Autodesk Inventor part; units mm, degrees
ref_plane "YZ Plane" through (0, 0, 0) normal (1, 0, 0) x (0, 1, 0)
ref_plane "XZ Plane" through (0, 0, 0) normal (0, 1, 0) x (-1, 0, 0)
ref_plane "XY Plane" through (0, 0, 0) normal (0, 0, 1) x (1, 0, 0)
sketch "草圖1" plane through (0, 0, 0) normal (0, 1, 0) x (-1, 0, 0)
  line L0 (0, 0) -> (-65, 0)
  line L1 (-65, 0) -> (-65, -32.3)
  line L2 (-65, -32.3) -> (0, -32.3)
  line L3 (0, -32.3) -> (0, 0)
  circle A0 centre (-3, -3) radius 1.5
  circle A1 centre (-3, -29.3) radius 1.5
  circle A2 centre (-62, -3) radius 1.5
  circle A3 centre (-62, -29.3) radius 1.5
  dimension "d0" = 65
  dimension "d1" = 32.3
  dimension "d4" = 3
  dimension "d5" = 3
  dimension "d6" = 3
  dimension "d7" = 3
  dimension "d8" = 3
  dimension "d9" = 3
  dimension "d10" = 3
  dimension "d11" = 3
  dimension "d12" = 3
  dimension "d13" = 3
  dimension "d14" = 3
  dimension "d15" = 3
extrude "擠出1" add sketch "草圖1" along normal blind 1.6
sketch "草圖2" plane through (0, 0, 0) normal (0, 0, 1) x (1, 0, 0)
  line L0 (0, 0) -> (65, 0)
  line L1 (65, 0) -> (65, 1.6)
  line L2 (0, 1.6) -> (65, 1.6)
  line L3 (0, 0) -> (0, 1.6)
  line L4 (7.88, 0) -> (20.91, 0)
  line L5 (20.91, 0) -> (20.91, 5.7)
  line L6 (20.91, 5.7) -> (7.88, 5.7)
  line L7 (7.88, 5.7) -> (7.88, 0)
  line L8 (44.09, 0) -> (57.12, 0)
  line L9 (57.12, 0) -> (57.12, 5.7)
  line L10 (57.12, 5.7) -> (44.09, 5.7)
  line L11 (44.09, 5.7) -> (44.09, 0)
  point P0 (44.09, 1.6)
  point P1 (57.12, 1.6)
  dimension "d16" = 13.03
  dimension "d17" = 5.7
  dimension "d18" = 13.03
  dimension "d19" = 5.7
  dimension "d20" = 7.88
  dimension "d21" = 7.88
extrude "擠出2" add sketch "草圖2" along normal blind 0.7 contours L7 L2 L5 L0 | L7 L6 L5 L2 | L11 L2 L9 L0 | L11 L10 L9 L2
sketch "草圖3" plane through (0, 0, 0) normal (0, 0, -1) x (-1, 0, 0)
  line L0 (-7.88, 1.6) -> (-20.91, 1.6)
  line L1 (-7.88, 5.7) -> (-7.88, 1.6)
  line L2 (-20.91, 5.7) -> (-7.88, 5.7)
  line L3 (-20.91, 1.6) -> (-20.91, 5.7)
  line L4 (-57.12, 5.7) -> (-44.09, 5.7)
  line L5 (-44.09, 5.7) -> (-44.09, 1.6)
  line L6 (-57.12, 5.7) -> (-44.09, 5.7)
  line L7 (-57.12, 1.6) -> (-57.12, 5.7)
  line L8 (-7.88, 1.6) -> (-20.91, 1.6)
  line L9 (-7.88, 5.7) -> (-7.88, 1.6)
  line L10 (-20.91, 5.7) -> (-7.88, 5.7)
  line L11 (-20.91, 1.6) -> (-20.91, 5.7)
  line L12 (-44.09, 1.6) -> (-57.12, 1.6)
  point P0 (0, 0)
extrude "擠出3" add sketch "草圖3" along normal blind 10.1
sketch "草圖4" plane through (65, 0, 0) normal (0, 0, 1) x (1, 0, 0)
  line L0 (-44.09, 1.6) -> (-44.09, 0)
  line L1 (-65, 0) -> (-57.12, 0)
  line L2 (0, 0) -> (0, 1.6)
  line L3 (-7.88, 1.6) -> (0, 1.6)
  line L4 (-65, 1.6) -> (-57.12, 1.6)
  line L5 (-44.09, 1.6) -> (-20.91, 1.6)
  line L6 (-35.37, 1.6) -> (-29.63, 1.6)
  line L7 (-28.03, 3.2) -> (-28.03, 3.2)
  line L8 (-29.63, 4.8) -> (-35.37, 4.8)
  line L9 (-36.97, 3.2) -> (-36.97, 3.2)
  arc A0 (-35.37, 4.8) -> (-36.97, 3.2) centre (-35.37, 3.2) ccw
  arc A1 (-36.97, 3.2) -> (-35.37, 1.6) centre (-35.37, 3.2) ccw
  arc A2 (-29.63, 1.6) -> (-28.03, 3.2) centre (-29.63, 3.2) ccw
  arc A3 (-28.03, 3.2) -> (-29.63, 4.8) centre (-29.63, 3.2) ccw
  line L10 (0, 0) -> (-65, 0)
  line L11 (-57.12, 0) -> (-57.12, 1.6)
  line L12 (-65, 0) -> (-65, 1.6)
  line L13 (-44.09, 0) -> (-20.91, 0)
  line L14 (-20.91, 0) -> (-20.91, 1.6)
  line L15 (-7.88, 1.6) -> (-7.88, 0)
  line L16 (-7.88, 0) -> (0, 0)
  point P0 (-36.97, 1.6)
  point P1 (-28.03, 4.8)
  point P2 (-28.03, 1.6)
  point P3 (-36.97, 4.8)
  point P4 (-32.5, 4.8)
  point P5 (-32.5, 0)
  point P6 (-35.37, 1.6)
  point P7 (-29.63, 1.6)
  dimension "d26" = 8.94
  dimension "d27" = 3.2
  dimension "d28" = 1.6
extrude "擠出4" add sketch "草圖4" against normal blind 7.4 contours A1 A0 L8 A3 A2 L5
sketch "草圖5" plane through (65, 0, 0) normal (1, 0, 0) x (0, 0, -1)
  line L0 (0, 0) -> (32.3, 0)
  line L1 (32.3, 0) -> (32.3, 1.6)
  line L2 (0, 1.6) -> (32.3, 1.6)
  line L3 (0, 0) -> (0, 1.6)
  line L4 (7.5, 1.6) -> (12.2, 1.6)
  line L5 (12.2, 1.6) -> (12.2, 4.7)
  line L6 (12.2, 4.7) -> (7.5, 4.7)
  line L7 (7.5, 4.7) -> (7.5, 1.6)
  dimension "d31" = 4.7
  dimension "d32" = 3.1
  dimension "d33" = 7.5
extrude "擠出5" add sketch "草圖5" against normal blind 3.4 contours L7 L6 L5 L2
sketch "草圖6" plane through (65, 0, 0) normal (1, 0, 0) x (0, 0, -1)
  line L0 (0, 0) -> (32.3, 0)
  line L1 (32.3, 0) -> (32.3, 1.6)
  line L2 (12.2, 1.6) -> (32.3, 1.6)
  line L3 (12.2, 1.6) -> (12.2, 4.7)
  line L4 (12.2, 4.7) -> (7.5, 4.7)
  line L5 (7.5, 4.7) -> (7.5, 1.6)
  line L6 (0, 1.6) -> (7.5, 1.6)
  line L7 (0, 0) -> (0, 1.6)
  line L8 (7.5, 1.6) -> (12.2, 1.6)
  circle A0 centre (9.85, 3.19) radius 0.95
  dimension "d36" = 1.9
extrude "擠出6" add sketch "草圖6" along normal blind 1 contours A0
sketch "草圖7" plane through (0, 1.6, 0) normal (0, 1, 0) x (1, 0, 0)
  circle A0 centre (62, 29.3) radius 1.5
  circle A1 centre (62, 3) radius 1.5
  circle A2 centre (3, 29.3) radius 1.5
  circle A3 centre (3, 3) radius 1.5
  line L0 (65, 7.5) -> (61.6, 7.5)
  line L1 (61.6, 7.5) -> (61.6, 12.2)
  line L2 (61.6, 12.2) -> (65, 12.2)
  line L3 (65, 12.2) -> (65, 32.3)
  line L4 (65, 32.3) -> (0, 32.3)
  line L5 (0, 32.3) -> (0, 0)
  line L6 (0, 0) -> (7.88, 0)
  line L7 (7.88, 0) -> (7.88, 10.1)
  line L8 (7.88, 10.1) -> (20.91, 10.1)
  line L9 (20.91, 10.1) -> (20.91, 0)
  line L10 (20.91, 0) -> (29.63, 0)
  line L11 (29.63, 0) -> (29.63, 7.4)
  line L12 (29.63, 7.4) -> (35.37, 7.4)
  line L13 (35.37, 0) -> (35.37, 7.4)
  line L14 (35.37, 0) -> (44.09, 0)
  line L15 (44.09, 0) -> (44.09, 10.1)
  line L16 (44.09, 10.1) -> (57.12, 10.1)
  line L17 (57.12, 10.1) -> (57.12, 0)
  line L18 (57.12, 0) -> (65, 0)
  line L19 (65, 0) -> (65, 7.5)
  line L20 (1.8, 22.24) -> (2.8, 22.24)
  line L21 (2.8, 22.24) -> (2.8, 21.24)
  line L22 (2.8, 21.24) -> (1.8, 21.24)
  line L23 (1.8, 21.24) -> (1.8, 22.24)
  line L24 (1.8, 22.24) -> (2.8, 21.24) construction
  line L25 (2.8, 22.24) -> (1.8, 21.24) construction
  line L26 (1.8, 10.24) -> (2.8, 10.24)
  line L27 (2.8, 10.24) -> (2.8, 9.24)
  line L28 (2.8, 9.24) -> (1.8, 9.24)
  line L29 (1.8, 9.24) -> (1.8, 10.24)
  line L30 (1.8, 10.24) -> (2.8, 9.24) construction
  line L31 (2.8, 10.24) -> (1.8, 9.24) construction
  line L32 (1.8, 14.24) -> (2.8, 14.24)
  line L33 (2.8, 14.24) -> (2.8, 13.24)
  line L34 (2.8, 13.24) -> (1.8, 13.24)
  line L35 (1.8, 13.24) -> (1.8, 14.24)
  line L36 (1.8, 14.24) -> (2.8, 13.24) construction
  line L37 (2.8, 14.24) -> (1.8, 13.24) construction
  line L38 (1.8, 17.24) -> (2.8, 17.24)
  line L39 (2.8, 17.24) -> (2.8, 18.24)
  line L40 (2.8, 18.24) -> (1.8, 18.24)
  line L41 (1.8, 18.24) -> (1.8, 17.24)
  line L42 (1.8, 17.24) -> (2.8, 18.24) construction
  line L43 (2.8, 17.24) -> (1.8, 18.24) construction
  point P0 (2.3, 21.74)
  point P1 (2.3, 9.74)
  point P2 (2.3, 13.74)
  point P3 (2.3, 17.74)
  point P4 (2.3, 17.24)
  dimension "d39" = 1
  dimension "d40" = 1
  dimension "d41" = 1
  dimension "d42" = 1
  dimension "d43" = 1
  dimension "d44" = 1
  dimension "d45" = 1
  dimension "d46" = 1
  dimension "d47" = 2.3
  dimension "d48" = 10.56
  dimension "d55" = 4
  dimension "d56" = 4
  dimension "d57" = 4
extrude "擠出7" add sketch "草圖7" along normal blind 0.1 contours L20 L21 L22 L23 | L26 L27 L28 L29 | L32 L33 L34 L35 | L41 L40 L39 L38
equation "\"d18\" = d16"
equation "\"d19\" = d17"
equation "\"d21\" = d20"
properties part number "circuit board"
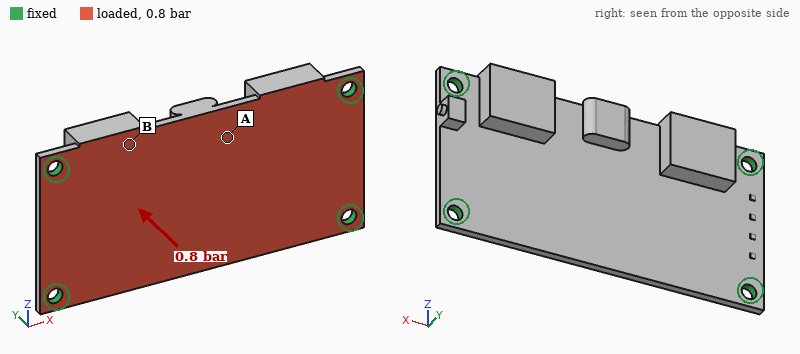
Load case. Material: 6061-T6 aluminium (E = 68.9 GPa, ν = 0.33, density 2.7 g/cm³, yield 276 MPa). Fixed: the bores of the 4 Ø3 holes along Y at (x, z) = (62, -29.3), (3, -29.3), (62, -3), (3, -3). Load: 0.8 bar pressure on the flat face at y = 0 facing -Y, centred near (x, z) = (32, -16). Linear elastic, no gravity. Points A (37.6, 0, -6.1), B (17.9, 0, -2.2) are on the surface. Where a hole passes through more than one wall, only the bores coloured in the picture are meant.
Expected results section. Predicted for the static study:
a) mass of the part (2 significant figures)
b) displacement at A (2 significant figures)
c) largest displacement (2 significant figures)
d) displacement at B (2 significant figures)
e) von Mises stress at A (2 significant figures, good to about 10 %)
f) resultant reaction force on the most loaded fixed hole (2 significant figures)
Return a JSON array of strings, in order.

["13 g", "0.095 mm", "0.12 mm", "0.056 mm", "26 MPa", "42 N"]
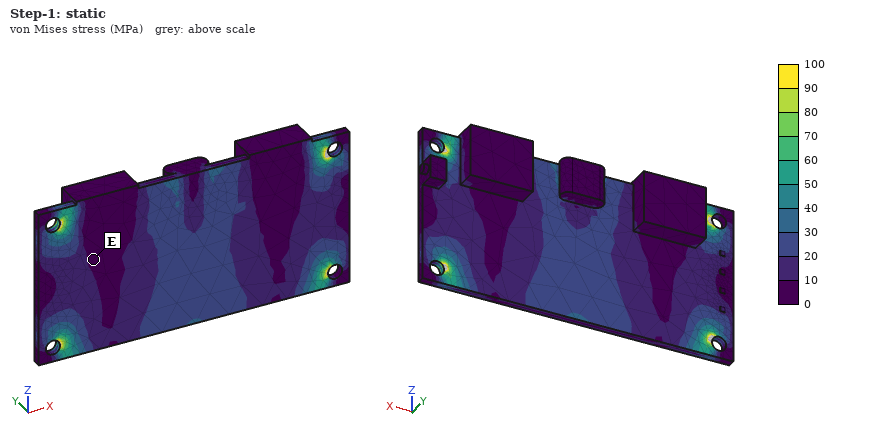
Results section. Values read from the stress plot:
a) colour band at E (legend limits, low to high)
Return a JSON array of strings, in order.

["0 to 10 MPa"]
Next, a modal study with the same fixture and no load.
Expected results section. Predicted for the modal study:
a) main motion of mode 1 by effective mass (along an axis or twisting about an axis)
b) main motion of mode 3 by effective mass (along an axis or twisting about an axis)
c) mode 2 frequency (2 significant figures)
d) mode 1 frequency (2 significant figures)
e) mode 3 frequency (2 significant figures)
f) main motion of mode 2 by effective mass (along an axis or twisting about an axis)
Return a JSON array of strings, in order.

["along Y", "twisting about Z", "4100 Hz", "2100 Hz", "5900 Hz", "twisting about X"]
